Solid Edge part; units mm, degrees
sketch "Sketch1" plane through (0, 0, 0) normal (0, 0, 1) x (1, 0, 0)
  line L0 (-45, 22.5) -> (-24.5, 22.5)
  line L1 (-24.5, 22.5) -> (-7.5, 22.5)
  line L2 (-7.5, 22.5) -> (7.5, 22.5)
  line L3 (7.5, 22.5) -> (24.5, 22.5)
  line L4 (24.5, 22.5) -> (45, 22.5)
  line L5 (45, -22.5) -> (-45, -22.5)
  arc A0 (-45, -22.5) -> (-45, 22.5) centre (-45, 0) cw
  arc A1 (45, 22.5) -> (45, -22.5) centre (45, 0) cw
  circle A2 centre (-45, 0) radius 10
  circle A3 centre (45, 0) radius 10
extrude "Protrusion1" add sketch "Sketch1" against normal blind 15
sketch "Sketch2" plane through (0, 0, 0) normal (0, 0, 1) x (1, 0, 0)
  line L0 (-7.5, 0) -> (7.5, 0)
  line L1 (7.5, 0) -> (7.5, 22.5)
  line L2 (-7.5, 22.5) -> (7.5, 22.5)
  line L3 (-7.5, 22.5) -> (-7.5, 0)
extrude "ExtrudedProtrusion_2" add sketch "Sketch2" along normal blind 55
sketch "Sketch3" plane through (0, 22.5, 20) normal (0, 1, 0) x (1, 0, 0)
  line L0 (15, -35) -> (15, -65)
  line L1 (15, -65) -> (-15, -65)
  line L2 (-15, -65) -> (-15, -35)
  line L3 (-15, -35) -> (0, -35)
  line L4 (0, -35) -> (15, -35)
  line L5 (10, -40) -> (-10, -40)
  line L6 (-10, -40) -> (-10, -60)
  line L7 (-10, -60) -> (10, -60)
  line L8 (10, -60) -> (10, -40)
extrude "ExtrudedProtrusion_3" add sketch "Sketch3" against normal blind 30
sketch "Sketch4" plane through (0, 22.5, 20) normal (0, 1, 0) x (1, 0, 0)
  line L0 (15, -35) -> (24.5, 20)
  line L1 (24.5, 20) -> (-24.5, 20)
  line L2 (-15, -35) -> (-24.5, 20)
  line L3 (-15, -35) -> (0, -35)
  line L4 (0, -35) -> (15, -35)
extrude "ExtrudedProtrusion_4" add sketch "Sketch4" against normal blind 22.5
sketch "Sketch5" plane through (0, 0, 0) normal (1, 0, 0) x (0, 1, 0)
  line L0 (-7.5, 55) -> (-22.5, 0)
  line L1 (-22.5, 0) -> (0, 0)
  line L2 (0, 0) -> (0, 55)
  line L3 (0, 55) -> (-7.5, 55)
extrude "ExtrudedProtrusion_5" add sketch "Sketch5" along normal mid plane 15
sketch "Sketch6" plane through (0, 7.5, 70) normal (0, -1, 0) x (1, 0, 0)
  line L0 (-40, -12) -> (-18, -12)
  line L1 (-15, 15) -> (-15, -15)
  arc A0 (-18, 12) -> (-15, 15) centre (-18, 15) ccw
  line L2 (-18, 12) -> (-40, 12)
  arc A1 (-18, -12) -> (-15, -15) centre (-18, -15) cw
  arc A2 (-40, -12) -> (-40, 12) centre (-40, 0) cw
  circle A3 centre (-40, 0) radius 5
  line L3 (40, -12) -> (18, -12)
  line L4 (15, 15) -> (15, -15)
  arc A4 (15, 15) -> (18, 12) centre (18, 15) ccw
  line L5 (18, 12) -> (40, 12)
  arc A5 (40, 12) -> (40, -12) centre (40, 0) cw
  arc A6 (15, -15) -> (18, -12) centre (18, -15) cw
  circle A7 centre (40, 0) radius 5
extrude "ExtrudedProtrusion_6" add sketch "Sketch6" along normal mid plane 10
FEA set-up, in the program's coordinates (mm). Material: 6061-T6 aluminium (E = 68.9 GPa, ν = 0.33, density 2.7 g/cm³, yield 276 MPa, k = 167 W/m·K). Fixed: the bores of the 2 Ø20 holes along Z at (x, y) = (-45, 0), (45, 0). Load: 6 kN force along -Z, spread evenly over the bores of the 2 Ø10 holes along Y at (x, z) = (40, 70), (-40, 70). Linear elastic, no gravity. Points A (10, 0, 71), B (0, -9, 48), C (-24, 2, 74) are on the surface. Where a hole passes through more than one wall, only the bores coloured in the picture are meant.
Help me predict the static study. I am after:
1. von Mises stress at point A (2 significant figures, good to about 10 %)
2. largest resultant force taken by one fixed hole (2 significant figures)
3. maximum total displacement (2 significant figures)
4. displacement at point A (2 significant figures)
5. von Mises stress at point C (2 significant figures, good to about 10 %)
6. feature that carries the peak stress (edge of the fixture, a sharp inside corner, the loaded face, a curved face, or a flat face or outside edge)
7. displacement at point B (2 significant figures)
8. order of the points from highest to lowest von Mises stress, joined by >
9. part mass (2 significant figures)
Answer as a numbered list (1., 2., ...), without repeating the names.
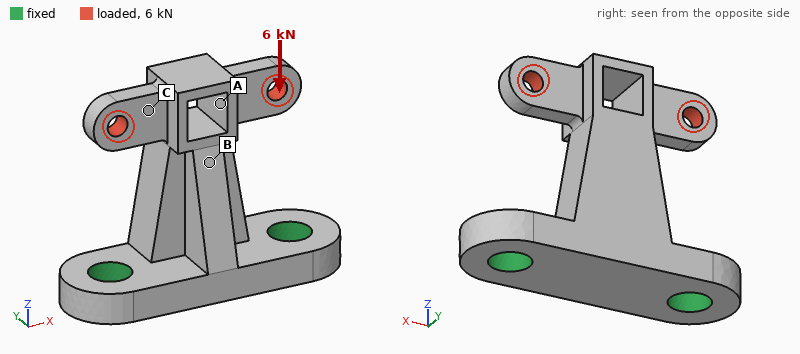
1. 18 MPa
2. 3.2 kN
3. 100 µm
4. 22 µm
5. 32 MPa
6. a curved face
7. 16 µm
8. C > A > B
9. 450 g
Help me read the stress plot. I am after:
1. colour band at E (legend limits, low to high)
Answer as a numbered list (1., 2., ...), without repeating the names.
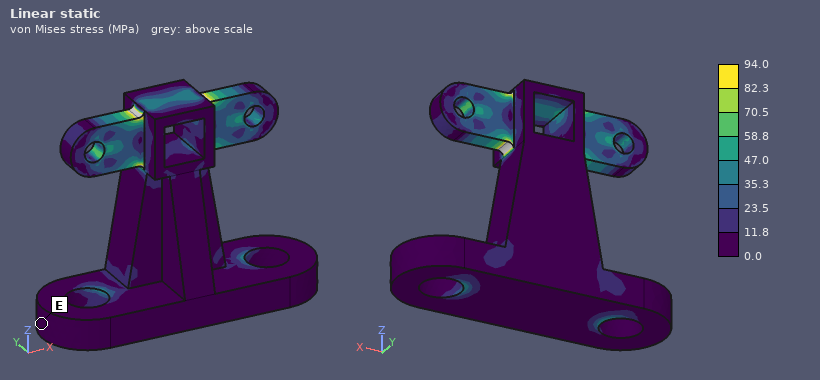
1. 0.0 to 11.8 MPa
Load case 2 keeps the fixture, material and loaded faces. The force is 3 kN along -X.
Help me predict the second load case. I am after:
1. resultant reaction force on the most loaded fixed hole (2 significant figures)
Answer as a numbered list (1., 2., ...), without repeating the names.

1. 4.0 kN
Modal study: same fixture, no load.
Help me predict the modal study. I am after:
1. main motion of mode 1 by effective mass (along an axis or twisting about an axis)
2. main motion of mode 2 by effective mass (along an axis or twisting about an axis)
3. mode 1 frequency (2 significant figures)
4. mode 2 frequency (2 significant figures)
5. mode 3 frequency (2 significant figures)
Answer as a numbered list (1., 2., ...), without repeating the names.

1. along Y
2. along X
3. 1700 Hz
4. 2400 Hz
5. 3400 Hz
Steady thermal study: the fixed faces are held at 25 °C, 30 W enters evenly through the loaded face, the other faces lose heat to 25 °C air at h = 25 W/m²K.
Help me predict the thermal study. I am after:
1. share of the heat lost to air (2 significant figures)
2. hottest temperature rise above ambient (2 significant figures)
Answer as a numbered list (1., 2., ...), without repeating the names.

1. 21 %
2. 27 K
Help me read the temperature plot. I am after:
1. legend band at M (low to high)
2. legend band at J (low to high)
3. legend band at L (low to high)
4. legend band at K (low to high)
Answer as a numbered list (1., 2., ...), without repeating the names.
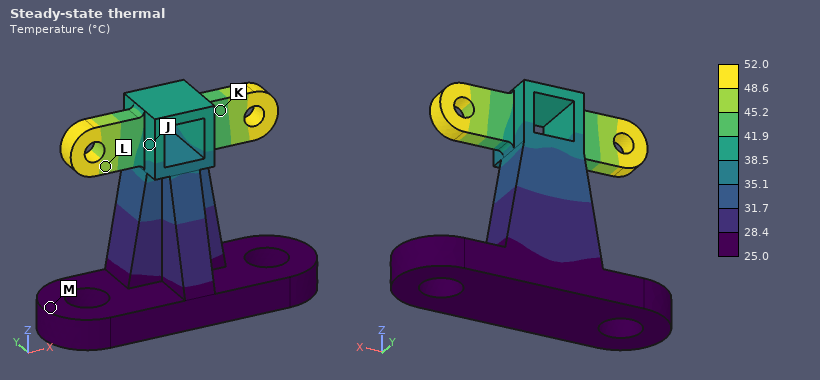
1. 25.0 to 28.4 °C
2. 38.5 to 41.9 °C
3. 45.2 to 48.6 °C
4. 41.9 to 45.2 °C
